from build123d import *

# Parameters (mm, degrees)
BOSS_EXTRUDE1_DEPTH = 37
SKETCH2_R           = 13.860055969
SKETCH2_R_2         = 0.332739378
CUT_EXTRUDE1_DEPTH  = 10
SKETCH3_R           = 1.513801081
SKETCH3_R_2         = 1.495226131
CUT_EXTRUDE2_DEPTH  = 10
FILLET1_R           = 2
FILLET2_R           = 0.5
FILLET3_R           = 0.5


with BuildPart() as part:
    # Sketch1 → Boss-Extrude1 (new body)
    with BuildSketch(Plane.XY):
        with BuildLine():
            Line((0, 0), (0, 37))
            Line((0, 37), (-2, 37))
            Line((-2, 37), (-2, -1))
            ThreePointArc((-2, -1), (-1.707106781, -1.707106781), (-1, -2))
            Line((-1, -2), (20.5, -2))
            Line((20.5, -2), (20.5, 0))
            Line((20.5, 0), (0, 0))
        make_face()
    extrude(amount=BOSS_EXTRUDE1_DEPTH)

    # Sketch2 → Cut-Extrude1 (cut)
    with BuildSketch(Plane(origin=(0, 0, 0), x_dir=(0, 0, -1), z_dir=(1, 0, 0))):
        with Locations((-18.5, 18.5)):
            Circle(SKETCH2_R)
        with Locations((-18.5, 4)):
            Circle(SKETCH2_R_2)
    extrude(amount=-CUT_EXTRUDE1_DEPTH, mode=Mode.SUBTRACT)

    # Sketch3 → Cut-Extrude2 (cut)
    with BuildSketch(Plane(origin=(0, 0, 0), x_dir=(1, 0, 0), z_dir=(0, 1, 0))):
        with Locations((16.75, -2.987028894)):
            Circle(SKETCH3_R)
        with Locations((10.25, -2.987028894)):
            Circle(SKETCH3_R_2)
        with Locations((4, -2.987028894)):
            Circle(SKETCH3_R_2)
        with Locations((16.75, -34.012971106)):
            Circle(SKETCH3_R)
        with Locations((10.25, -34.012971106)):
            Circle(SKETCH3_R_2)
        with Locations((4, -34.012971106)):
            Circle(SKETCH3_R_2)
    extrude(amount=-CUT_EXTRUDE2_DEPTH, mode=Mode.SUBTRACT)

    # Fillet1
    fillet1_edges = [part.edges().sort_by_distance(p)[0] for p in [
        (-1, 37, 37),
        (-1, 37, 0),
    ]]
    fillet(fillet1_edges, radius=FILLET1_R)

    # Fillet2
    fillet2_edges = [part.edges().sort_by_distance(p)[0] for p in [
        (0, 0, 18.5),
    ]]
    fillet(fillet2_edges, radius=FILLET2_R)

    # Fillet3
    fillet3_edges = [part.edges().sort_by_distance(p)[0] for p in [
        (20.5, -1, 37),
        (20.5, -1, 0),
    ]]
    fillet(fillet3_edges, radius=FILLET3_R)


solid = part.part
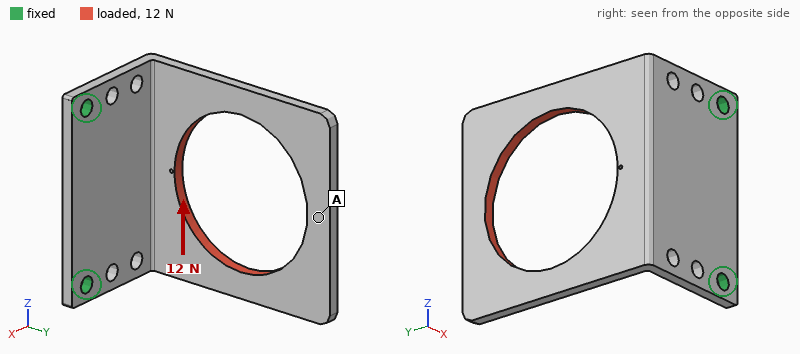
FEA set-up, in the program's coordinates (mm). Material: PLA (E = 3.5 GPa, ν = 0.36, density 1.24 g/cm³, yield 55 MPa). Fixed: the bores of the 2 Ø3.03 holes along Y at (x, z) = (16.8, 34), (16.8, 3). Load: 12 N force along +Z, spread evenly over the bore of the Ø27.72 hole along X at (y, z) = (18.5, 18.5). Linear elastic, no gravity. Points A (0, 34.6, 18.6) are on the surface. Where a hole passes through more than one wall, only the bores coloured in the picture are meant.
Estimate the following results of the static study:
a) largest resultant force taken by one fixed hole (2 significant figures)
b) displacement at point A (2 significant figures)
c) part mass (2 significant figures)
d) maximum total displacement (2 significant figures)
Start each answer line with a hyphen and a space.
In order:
- 12 N
- 0.53 mm
- 3.8 g
- 0.62 mm
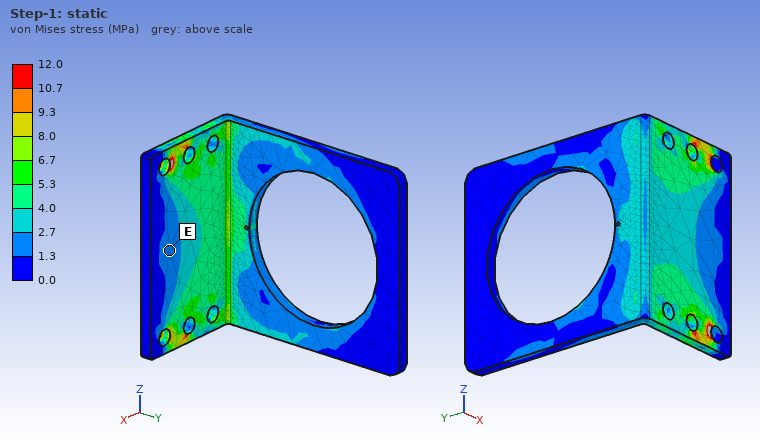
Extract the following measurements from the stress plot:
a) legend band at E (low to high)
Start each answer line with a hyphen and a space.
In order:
- 1.3 to 2.7 MPa
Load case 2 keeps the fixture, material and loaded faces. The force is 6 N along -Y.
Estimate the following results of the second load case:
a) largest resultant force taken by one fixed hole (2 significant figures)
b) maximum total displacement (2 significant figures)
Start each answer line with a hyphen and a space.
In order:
- 3.0 N
- 0.59 mm
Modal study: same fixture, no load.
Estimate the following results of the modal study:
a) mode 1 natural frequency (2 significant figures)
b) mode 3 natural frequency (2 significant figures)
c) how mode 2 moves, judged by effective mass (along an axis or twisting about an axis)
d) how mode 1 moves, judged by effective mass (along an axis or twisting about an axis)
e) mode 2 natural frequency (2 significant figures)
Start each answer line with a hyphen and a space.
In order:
- 220 Hz
- 730 Hz
- along Z
- along X
- 510 Hz
